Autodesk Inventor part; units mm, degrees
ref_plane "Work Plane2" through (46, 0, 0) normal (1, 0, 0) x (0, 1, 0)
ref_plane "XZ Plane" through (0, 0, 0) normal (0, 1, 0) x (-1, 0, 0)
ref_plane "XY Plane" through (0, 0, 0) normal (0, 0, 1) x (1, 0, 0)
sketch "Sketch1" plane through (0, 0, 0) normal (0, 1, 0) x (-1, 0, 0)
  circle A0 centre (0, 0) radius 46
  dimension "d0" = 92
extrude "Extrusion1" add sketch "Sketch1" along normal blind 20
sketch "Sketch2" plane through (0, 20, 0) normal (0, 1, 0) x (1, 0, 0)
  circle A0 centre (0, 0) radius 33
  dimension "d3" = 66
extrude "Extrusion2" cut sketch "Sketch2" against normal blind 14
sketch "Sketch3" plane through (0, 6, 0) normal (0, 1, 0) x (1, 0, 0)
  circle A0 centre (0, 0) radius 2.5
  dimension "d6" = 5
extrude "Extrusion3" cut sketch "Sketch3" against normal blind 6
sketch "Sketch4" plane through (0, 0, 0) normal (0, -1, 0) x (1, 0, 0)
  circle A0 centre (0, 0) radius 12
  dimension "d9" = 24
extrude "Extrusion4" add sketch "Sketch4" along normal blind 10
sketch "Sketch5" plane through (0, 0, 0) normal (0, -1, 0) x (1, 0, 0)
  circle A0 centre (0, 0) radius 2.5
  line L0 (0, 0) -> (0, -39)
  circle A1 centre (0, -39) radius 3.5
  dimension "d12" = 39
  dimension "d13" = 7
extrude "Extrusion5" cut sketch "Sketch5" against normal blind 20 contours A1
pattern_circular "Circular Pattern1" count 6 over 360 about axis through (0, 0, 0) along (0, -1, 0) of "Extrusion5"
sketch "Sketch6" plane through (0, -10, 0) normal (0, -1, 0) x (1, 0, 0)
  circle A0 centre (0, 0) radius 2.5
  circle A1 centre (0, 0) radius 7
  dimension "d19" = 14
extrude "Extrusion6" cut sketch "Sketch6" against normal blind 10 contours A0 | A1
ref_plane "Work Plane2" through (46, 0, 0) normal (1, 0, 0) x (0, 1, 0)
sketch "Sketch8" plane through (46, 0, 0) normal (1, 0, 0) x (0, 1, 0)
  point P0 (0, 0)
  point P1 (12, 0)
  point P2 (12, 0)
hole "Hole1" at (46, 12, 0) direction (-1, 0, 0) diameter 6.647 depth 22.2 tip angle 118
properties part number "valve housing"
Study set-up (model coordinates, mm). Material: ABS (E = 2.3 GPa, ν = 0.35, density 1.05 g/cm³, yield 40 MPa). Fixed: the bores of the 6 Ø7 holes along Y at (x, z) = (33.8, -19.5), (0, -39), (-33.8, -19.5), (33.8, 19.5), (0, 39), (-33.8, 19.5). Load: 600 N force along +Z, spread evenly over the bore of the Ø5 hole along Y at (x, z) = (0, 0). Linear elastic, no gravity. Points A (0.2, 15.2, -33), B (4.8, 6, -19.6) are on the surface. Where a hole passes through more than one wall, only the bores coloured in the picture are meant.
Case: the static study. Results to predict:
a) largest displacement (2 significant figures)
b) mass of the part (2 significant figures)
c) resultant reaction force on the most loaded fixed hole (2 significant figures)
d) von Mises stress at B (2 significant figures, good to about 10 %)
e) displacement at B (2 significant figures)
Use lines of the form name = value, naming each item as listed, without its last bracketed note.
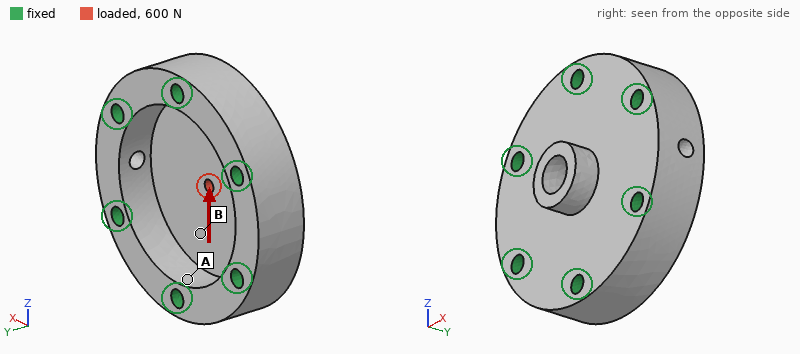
largest displacement = 34 µm
mass of the part = 87 g
resultant reaction force on the most loaded fixed hole = 150 N
von Mises stress at B = 1.5 MPa
displacement at B = 11 µm
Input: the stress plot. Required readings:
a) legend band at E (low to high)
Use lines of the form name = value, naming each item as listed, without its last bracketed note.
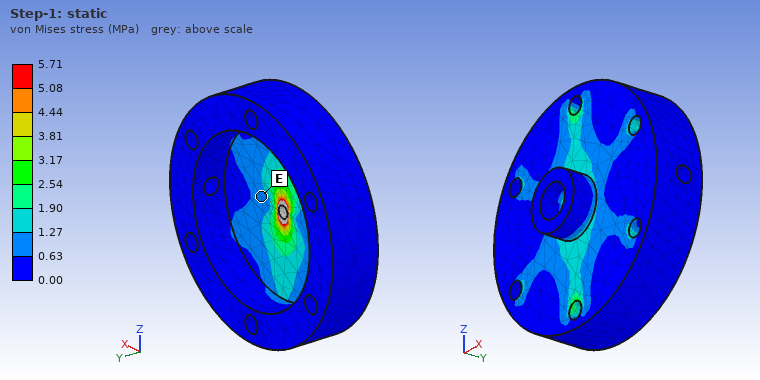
legend band at E = 0.63 to 1.27 MPa
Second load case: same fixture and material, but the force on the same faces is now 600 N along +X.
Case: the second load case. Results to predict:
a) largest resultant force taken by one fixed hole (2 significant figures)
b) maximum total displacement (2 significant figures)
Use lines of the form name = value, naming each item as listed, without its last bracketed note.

largest resultant force taken by one fixed hole = 140 N
maximum total displacement = 34 µm
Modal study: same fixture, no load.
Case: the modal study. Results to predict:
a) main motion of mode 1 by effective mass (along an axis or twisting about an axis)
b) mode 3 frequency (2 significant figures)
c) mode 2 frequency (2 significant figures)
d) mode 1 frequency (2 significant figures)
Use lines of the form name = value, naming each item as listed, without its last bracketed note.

main motion of mode 1 by effective mass = along Y
mode 3 frequency = 5200 Hz
mode 2 frequency = 5200 Hz
mode 1 frequency = 3000 Hz
